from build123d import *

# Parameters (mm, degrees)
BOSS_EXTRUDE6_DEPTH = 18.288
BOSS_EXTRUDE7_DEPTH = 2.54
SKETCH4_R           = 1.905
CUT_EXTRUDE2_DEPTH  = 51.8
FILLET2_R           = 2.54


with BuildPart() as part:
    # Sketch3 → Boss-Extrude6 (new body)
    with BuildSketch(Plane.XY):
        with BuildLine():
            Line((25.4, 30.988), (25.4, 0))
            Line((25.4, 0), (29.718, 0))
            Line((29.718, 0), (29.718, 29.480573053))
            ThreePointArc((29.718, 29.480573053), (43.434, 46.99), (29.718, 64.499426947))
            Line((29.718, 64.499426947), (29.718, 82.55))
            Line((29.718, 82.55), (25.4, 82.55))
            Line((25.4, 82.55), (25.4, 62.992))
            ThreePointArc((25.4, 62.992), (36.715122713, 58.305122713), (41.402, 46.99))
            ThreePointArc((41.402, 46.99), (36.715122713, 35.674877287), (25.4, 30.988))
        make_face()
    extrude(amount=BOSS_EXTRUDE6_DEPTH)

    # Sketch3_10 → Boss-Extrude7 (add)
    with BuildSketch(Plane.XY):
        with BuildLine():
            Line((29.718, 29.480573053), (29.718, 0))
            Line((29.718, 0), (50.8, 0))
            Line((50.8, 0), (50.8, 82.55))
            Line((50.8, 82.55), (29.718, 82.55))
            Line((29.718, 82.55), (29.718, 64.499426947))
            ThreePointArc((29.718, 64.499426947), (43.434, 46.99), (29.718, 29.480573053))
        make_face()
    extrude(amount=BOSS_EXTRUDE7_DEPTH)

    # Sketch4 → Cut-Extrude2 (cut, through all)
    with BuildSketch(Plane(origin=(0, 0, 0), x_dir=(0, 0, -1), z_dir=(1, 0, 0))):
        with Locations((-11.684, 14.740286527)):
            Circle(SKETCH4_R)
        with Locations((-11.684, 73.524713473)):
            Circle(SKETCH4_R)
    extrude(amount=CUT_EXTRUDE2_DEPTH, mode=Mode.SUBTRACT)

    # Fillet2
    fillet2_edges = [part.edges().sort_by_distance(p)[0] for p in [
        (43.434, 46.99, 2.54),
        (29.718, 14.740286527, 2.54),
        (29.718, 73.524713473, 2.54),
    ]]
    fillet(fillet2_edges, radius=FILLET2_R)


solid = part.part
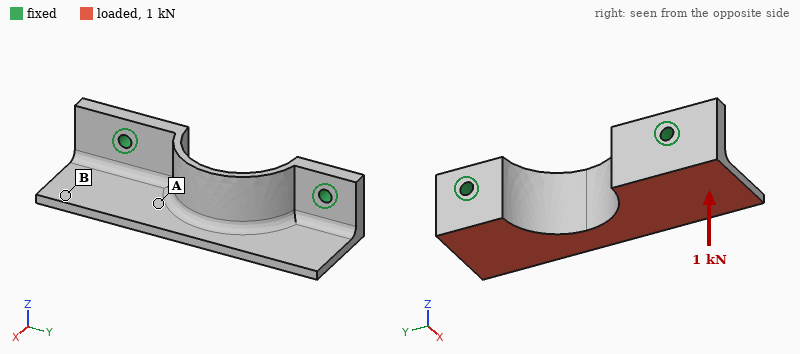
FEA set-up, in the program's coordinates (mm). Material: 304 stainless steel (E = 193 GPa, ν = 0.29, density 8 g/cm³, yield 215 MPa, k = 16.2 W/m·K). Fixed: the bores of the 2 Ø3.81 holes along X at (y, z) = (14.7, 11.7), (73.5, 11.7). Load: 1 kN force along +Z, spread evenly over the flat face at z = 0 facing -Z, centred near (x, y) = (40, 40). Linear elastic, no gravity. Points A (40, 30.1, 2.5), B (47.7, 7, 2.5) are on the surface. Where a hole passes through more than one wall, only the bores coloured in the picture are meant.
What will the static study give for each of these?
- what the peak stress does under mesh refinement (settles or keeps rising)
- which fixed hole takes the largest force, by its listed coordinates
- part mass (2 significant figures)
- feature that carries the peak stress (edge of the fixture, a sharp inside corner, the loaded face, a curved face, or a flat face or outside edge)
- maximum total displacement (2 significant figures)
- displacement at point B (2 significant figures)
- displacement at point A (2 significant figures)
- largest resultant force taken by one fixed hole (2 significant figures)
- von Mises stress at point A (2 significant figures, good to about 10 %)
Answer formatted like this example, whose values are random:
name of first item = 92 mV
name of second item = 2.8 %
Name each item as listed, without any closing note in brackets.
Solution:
what the peak stress does under mesh refinement = keeps rising
which fixed hole takes the largest force, by its listed coordinates = (14.7, 11.7)
part mass = 74 g
feature that carries the peak stress = edge of the fixture
maximum total displacement = 77 µm
displacement at point B = 63 µm
displacement at point A = 29 µm
largest resultant force taken by one fixed hole = 540 N
von Mises stress at point A = 33 MPa
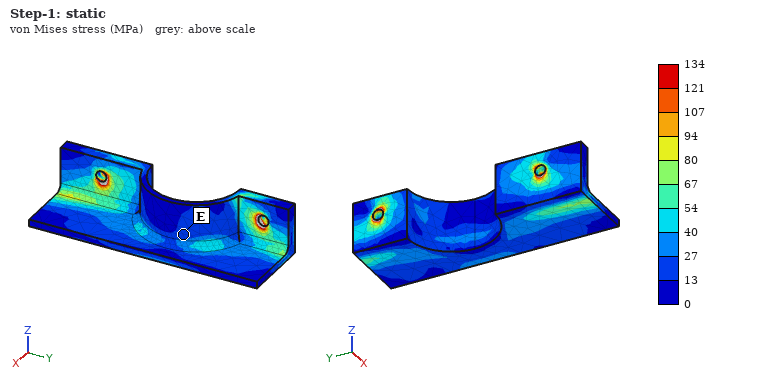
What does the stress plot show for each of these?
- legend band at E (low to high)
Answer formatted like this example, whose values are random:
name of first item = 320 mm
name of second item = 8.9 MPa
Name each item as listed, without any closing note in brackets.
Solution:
legend band at E = 13 to 27 MPa
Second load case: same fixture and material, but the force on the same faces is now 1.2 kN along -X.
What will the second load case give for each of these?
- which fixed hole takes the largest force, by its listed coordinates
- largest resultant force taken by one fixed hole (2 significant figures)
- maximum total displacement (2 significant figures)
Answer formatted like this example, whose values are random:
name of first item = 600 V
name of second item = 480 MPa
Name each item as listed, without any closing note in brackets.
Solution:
which fixed hole takes the largest force, by its listed coordinates = (14.7, 11.7)
largest resultant force taken by one fixed hole = 700 N
maximum total displacement = 43 µm
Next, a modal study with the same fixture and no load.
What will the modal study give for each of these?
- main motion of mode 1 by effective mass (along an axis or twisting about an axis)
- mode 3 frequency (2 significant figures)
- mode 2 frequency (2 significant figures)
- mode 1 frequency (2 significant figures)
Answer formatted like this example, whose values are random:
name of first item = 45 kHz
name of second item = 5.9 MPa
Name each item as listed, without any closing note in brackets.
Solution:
main motion of mode 1 by effective mass = along Z
mode 3 frequency = 6300 Hz
mode 2 frequency = 4700 Hz
mode 1 frequency = 3700 Hz
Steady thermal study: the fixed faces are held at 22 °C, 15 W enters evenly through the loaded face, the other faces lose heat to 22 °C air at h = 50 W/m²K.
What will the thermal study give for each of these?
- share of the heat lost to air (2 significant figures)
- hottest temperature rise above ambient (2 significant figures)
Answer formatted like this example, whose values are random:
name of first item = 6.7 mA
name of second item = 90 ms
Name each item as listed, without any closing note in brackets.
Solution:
share of the heat lost to air = 51 %
hottest temperature rise above ambient = 57 K
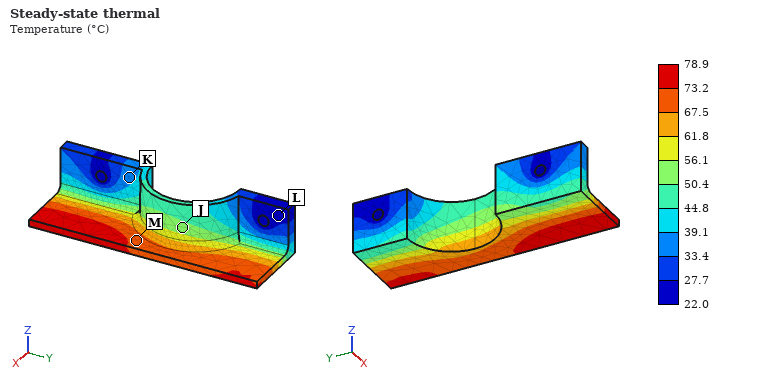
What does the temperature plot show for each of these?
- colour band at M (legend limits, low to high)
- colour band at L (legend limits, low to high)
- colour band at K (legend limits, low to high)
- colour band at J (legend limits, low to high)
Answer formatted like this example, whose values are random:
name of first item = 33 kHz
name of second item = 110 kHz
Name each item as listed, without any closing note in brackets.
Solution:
colour band at M = 67.5 to 73.2 °C
colour band at L = 22.0 to 27.7 °C
colour band at K = 33.4 to 39.1 °C
colour band at J = 50.4 to 56.1 °C
